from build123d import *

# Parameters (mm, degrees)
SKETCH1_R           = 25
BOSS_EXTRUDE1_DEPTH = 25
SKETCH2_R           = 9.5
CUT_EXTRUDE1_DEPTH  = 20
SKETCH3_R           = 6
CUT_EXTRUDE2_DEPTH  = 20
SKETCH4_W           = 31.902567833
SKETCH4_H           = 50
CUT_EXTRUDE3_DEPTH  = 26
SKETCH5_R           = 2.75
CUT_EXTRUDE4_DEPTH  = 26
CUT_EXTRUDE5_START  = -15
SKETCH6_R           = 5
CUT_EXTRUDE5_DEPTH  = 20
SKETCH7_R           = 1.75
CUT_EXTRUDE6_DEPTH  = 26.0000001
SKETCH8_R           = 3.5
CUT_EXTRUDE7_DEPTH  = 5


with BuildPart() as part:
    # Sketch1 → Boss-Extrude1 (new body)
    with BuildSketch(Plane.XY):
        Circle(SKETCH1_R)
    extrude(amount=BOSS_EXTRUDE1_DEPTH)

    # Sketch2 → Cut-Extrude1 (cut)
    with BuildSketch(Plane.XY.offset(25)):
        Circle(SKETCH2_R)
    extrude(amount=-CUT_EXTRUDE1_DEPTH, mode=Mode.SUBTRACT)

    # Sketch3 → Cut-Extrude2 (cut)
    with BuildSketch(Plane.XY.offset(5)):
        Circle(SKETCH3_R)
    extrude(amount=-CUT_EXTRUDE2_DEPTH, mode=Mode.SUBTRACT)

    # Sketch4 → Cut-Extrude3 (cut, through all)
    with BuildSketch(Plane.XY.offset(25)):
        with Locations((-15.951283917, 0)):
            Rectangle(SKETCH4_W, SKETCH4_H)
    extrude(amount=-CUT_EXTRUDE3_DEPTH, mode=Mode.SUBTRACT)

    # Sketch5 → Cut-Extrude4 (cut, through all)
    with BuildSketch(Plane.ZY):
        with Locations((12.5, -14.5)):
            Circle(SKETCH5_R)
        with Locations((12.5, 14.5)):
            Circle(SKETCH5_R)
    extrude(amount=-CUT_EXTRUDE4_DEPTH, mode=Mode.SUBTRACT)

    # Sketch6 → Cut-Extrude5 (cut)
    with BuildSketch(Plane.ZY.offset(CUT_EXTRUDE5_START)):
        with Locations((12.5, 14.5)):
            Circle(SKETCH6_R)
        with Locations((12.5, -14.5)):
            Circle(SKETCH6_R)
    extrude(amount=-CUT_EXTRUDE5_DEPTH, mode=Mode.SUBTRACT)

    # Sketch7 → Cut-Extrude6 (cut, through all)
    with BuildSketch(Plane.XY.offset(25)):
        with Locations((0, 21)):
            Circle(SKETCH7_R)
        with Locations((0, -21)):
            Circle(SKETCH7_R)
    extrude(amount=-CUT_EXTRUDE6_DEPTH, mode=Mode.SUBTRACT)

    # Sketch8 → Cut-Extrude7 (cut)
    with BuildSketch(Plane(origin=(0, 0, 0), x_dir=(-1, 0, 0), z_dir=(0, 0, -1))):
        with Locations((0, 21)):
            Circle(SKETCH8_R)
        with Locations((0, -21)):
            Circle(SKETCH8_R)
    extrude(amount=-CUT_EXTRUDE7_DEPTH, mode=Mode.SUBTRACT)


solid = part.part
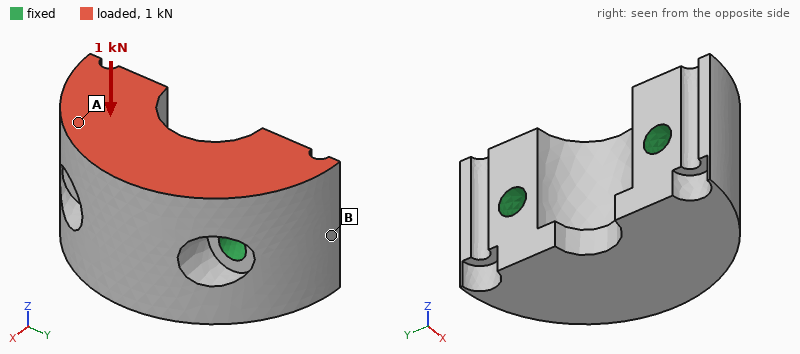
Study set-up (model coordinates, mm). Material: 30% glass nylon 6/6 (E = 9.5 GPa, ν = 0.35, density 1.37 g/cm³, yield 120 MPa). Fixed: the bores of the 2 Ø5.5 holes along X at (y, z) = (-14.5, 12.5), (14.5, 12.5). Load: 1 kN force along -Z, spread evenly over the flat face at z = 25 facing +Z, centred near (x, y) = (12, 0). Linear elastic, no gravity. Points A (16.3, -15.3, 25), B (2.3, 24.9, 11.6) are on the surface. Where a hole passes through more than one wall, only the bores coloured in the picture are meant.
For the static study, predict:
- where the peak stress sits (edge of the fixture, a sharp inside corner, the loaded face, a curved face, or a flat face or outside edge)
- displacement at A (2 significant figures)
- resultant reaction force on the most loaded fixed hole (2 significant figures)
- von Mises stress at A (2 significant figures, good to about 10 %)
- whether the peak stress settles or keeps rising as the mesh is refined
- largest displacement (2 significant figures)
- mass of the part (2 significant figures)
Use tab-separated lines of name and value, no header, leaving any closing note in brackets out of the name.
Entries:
where the peak stress sits	edge of the fixture
displacement at A	5.4 µm
resultant reaction force on the most loaded fixed hole	500 N
von Mises stress at A	2.0 MPa
whether the peak stress settles or keeps rising as the mesh is refined	keeps rising
largest displacement	10 µm
mass of the part	27 g
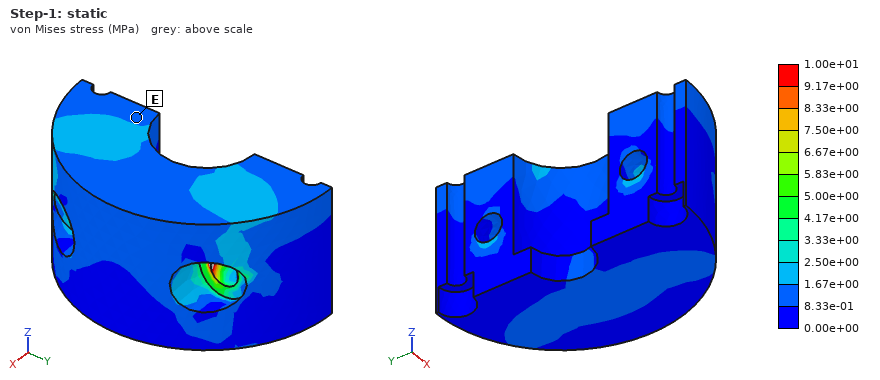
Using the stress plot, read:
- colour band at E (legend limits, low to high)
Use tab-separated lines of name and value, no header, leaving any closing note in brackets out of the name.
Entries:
colour band at E	8.33e-01 to 1.67e+00 MPa
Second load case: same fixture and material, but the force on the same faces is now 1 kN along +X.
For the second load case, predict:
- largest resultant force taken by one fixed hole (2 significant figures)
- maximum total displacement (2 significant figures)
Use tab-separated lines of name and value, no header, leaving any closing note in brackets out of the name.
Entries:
largest resultant force taken by one fixed hole	510 N
maximum total displacement	23 µm
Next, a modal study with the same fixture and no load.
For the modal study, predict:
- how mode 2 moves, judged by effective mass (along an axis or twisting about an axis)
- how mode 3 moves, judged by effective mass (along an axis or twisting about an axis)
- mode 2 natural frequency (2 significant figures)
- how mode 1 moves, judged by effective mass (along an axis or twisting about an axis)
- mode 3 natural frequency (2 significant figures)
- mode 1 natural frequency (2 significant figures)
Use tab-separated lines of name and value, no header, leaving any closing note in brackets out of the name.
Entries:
how mode 2 moves, judged by effective mass	along X
how mode 3 moves, judged by effective mass	twisting about X
mode 2 natural frequency	18 kHz
how mode 1 moves, judged by effective mass	along Z
mode 3 natural frequency	20 kHz
mode 1 natural frequency	12 kHz
